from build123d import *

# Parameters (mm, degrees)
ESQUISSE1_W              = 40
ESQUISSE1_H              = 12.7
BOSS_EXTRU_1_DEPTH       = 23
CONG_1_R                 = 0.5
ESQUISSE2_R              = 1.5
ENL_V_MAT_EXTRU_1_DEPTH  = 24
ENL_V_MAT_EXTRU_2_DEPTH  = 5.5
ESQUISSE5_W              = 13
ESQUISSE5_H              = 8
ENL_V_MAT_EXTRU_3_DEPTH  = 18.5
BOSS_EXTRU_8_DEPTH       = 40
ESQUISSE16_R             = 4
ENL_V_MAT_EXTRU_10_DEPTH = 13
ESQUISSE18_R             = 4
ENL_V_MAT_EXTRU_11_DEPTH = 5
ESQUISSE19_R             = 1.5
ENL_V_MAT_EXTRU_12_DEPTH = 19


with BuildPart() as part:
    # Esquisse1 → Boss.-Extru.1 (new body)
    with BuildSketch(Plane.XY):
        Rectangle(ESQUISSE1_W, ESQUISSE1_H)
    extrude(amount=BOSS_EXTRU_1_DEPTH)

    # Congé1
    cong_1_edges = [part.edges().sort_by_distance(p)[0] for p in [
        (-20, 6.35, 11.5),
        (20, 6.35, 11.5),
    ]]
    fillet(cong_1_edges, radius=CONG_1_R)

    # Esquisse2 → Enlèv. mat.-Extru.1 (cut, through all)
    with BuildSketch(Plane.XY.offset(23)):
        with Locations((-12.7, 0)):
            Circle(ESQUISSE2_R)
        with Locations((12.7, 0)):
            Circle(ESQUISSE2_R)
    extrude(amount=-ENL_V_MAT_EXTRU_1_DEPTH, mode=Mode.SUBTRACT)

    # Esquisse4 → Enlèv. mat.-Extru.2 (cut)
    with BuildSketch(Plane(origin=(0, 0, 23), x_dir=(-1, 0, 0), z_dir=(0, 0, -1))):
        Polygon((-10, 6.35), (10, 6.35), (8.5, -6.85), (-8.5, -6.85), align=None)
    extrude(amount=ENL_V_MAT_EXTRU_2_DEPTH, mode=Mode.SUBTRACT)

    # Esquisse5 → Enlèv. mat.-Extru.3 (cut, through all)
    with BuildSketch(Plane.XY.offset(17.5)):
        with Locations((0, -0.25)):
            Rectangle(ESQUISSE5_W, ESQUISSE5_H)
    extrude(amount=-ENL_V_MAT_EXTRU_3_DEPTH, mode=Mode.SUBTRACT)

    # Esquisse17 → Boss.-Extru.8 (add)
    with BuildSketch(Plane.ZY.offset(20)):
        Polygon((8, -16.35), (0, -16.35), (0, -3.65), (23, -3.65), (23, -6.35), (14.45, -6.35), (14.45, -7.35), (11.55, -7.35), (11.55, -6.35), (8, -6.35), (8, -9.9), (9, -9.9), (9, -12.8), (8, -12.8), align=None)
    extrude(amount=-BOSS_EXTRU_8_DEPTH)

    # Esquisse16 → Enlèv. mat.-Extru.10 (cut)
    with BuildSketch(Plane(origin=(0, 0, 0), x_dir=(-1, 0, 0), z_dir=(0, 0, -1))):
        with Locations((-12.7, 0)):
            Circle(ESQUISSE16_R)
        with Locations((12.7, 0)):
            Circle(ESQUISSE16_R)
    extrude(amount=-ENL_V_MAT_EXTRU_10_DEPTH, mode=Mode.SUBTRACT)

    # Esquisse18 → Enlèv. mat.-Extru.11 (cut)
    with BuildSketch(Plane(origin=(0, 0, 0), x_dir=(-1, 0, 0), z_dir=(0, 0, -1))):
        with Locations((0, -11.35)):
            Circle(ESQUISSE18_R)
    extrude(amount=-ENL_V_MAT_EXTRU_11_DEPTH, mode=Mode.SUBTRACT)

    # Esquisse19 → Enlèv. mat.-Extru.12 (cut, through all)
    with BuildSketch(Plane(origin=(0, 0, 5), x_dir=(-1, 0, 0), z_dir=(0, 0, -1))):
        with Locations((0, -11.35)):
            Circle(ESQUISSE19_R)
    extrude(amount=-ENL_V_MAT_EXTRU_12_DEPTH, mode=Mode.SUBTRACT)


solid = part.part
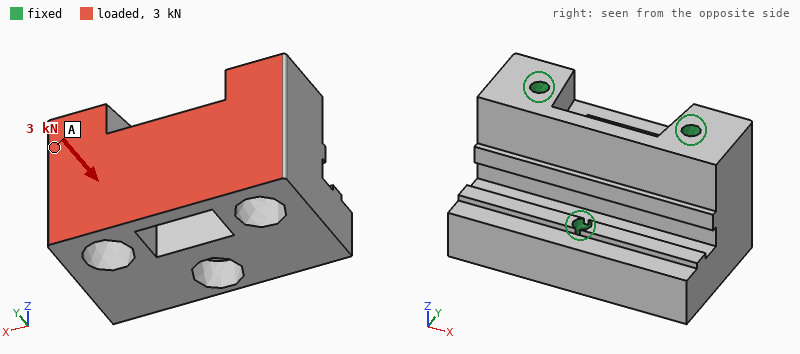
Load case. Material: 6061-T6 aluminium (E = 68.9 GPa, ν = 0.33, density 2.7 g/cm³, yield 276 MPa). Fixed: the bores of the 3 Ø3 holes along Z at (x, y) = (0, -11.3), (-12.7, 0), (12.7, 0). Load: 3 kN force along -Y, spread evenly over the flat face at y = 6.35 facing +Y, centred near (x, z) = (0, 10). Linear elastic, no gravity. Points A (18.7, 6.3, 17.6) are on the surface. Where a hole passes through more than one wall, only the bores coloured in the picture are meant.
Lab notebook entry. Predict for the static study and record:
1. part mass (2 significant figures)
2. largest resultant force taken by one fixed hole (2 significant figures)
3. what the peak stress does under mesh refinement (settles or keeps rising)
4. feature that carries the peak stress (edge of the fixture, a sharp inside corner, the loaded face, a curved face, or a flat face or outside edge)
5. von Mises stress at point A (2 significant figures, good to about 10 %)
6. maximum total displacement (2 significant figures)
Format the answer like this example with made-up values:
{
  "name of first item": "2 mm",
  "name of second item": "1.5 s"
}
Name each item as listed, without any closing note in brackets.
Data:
{
  "part mass": "29 g",
  "largest resultant force taken by one fixed hole": "1.1 kN",
  "what the peak stress does under mesh refinement": "keeps rising",
  "feature that carries the peak stress": "edge of the fixture",
  "von Mises stress at point A": "7.5 MPa",
  "maximum total displacement": "16 µm"
}
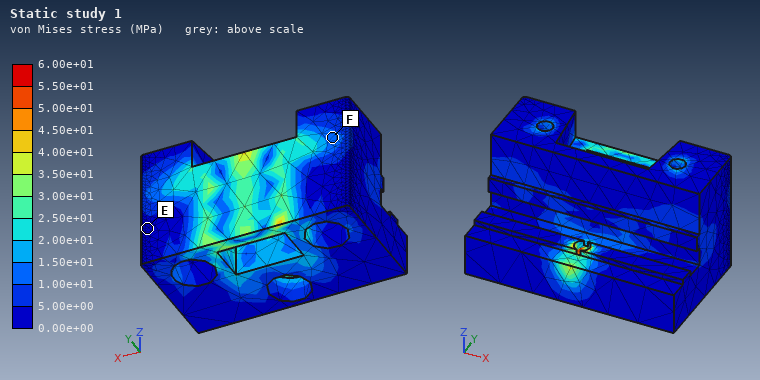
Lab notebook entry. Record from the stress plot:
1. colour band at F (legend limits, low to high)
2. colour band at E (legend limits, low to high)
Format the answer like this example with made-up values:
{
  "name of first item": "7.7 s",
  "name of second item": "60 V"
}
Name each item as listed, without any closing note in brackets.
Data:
{
  "colour band at F": "1.00e+01 to 1.50e+01 MPa",
  "colour band at E": "0.00e+00 to 5.00e+00 MPa"
}
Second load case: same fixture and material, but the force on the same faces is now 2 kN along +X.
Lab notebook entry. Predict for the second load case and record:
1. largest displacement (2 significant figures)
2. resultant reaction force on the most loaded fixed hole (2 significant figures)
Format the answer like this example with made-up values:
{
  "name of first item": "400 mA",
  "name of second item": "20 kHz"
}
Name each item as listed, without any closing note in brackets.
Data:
{
  "largest displacement": "9.8 µm",
  "resultant reaction force on the most loaded fixed hole": "1.1 kN"
}
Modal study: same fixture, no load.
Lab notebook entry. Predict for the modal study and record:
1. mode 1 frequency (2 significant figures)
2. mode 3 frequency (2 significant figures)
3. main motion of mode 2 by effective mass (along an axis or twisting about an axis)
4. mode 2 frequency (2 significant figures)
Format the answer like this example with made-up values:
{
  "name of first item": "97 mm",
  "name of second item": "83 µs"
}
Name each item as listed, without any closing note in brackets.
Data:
{
  "mode 1 frequency": "18 kHz",
  "mode 3 frequency": "28 kHz",
  "main motion of mode 2 by effective mass": "along Y",
  "mode 2 frequency": "19 kHz"
}
